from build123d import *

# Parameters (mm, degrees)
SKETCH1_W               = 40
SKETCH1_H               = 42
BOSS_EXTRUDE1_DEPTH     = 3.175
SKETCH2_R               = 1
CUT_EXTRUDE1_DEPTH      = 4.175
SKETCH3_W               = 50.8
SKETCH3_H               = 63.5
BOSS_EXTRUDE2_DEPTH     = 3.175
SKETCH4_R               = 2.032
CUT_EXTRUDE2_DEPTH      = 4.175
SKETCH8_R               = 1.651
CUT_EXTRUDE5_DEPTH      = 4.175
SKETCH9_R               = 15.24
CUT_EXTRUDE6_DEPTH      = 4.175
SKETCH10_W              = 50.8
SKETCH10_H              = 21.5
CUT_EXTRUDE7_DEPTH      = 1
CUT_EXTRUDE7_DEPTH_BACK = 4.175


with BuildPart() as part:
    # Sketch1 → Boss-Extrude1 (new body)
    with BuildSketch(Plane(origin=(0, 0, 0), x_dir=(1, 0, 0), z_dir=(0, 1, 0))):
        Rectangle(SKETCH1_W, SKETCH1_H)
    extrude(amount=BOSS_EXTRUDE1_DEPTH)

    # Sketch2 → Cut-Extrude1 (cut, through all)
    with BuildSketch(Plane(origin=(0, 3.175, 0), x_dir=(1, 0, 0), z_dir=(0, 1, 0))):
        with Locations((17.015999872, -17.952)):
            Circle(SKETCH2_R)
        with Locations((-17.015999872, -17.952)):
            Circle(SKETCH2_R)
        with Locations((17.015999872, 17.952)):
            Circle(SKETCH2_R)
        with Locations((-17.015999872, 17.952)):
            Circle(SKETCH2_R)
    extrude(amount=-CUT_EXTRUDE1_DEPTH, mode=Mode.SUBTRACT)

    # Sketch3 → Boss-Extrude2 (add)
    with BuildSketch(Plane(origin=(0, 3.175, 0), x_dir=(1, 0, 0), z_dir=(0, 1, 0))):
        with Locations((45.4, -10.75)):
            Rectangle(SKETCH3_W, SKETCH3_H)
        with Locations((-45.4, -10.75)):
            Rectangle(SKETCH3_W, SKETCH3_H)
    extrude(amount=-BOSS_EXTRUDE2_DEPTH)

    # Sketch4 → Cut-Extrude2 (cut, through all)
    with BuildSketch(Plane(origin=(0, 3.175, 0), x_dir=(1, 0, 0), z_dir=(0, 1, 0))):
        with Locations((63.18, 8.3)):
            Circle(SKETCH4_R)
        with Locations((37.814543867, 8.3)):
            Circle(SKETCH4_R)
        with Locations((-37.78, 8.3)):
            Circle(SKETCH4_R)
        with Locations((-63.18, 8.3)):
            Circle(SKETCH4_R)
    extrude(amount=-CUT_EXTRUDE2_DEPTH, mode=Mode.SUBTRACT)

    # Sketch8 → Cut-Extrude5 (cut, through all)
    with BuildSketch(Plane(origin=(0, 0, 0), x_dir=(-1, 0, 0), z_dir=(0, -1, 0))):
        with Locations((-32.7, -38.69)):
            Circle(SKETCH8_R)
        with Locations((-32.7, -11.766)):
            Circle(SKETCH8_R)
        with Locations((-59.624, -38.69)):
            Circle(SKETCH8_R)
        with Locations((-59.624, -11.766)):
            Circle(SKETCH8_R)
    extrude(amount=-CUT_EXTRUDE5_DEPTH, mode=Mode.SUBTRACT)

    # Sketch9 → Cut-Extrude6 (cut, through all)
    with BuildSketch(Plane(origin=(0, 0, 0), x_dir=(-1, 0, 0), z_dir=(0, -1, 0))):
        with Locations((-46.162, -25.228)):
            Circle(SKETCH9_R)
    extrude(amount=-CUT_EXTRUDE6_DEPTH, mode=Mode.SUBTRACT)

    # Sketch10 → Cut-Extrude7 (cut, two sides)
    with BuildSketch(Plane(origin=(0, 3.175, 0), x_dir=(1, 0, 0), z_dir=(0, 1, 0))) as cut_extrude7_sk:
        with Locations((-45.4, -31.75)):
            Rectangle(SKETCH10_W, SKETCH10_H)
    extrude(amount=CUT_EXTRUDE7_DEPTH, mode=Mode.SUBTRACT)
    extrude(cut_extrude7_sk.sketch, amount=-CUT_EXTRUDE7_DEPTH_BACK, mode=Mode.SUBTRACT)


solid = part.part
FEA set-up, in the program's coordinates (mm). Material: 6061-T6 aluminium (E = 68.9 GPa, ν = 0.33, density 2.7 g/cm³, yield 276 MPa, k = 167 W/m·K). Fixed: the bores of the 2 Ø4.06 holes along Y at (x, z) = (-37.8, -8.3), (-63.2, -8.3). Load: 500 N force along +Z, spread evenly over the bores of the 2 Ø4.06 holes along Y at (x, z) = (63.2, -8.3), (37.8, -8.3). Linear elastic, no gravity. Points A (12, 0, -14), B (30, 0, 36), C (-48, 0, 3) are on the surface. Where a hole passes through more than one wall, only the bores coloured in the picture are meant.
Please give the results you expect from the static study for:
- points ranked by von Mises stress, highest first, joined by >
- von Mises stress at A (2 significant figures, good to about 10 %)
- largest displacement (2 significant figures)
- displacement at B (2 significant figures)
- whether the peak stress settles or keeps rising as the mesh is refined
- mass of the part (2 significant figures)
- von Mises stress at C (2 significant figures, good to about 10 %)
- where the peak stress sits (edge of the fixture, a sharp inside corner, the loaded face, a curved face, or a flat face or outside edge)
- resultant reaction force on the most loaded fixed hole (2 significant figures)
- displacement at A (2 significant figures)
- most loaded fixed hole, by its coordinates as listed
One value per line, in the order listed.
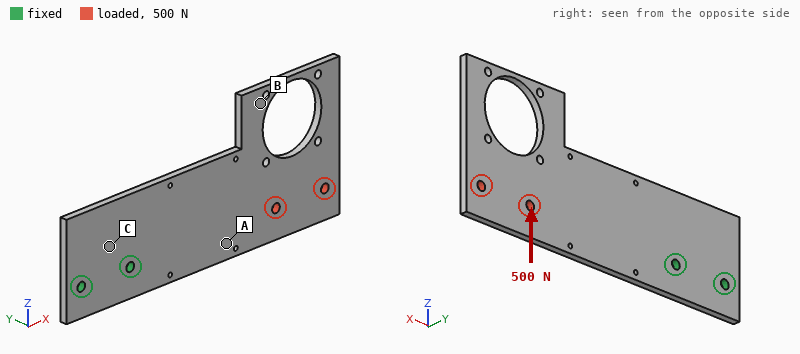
C > A > B
16 MPa
0.27 mm
0.17 mm
keeps rising
53 g
31 MPa
edge of the fixture
2.1 kN
0.097 mm
(-37.8, -8.3)
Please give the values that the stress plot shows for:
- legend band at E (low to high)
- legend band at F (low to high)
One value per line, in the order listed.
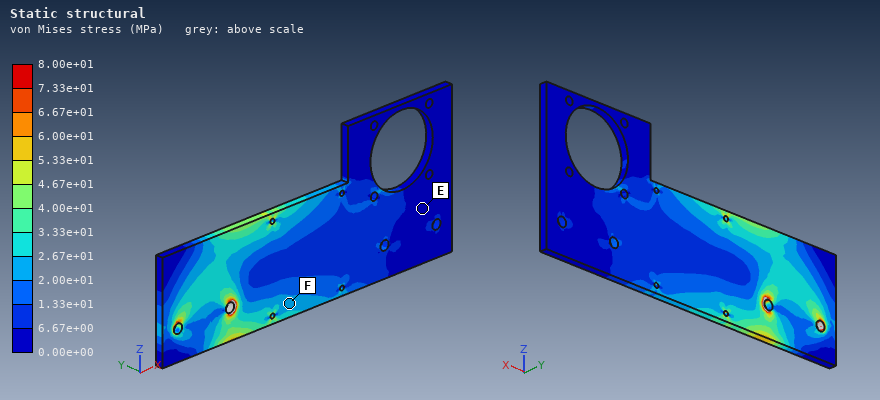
0.00e+00 to 6.67e+00 MPa
2.00e+01 to 2.67e+01 MPa
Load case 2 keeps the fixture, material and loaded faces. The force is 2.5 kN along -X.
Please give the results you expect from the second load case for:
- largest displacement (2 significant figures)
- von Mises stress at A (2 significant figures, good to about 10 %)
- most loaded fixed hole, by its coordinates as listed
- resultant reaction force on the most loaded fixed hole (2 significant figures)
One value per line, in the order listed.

98 µm
35 MPa
(-37.8, -8.3)
2.0 kN
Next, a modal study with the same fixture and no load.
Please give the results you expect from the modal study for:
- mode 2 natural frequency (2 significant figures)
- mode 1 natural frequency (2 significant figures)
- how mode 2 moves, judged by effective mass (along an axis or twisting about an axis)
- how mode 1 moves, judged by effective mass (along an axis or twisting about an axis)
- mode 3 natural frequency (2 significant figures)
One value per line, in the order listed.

670 Hz
200 Hz
twisting about X
along Y
1100 Hz
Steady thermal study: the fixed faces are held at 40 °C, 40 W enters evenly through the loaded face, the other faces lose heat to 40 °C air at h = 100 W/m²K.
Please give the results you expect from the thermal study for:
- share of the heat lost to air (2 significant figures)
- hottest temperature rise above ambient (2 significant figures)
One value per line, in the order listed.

82 %
70 K
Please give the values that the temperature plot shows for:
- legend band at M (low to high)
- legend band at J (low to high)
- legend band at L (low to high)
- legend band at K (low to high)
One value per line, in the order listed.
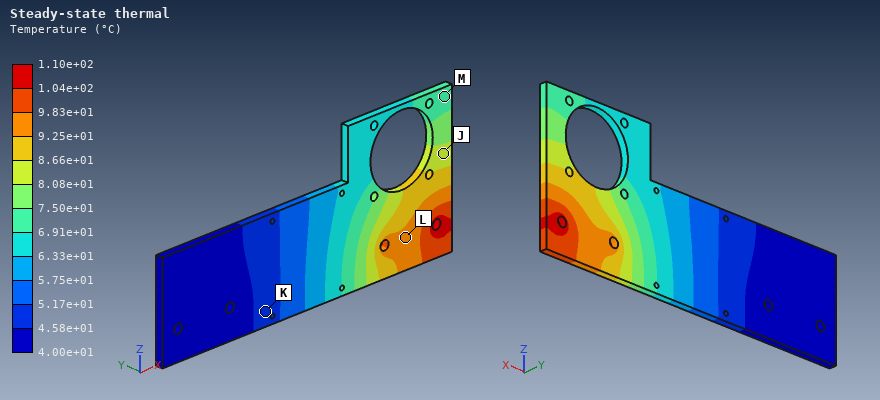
6.91e+01 to 7.50e+01 °C
8.08e+01 to 8.66e+01 °C
9.25e+01 to 9.83e+01 °C
4.58e+01 to 5.17e+01 °C
